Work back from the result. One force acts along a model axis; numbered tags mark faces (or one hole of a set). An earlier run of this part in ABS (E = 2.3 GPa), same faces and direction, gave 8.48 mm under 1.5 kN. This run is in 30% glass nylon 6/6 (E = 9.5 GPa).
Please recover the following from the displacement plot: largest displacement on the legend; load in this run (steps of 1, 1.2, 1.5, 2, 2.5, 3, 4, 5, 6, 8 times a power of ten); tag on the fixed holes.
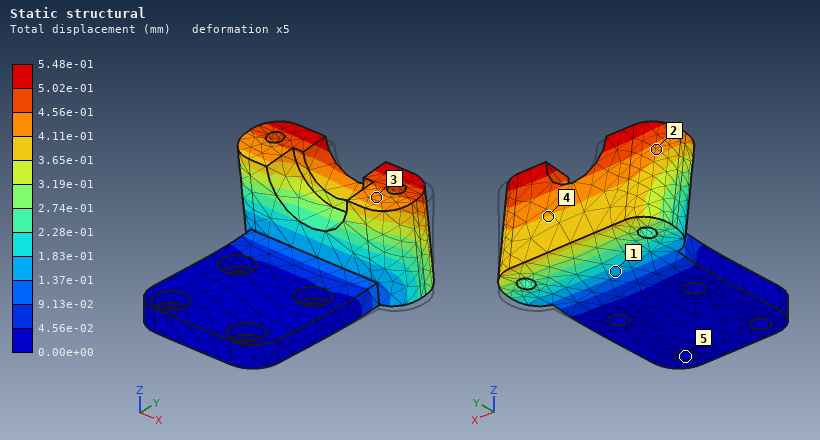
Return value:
5.48e-01 mm
400 N
5
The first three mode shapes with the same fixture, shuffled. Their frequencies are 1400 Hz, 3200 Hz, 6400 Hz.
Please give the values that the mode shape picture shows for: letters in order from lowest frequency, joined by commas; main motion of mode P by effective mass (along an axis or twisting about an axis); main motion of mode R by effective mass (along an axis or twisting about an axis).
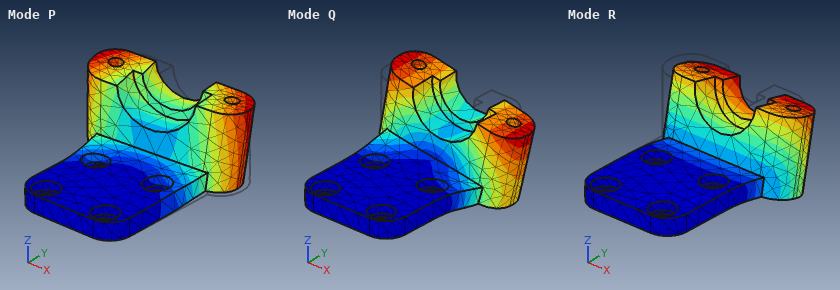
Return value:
R, Q, P
along X
along Z
